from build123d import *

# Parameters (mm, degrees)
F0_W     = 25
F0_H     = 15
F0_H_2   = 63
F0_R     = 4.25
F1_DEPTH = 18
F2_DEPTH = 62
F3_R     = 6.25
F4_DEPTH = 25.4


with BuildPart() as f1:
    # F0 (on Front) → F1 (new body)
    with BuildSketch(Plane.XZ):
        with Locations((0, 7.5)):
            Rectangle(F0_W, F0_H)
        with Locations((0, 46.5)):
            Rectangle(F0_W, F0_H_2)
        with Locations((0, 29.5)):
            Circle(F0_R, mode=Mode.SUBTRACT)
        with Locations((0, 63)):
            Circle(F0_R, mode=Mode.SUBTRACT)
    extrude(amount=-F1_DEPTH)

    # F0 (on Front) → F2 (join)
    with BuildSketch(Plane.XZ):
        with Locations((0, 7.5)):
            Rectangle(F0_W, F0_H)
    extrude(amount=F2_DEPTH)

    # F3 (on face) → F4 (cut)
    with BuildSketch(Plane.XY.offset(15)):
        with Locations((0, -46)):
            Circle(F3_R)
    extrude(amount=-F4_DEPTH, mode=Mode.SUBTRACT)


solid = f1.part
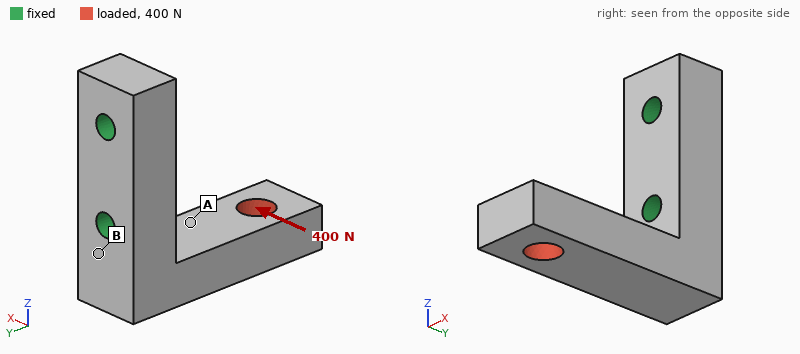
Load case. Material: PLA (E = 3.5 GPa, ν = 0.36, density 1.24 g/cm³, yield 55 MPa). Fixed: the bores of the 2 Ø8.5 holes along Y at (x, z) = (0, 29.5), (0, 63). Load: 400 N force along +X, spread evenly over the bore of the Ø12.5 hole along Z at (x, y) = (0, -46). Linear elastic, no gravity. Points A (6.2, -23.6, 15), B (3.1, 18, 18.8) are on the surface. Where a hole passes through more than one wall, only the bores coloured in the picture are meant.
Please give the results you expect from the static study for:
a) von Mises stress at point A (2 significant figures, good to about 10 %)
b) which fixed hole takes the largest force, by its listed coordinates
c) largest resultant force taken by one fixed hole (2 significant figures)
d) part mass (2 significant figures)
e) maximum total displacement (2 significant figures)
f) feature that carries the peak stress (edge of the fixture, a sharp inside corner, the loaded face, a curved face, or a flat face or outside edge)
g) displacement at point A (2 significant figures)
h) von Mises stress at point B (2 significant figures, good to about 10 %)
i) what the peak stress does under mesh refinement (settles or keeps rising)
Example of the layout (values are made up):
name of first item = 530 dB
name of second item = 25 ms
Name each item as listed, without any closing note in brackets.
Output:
von Mises stress at point A = 3.6 MPa
which fixed hole takes the largest force, by its listed coordinates = (0, 29.5)
largest resultant force taken by one fixed hole = 510 N
part mass = 68 g
maximum total displacement = 1.2 mm
feature that carries the peak stress = edge of the fixture
displacement at point A = 0.50 mm
von Mises stress at point B = 12 MPa
what the peak stress does under mesh refinement = keeps rising
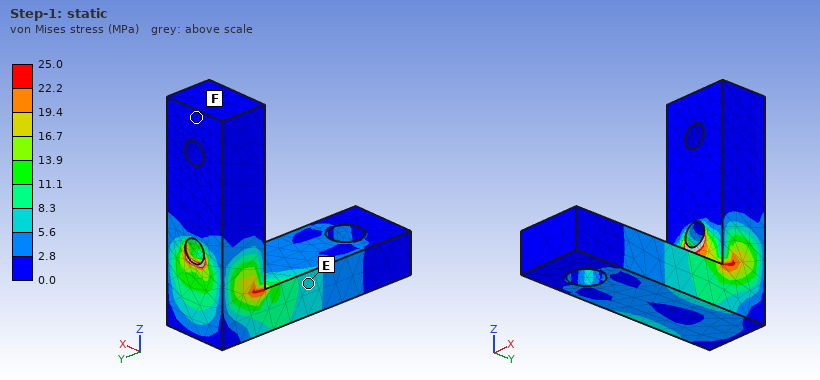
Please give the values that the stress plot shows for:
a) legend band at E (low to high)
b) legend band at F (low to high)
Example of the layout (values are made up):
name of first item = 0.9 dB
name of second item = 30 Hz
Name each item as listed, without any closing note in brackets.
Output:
legend band at E = 5.6 to 8.3 MPa
legend band at F = 0.0 to 2.8 MPa
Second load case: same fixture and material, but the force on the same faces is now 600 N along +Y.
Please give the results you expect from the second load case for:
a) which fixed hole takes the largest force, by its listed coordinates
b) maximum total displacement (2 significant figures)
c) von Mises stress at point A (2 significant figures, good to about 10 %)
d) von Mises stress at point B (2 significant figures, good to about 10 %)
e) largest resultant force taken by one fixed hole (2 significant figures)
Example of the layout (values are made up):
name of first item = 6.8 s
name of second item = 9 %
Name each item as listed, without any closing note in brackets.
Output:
which fixed hole takes the largest force, by its listed coordinates = (0, 29.5)
maximum total displacement = 0.29 mm
von Mises stress at point A = 1.6 MPa
von Mises stress at point B = 5.5 MPa
largest resultant force taken by one fixed hole = 650 N
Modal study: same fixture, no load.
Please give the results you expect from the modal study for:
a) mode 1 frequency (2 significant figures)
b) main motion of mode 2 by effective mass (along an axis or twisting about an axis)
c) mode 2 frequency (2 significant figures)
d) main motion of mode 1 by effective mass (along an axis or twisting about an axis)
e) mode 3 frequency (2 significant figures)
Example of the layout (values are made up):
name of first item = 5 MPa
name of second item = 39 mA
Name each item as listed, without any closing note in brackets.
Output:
mode 1 frequency = 700 Hz
main motion of mode 2 by effective mass = along X
mode 2 frequency = 830 Hz
main motion of mode 1 by effective mass = along Z
mode 3 frequency = 2600 Hz
